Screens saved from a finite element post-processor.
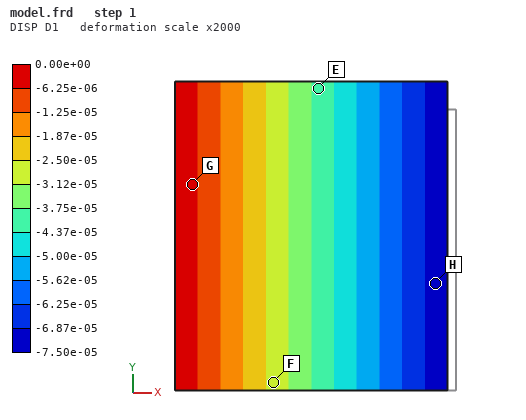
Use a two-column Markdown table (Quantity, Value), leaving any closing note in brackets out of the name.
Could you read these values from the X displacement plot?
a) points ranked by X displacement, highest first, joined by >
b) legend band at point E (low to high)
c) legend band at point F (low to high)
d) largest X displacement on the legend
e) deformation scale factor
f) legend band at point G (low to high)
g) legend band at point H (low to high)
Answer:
| Quantity | Value |
|---|---|
| points ranked by X displacement, highest first, joined by > | G > F > E > H |
| legend band at point E | -4.37e-05 to -3.75e-05 |
| legend band at point F | -3.12e-05 to -2.50e-05 |
| largest X displacement on the legend | 0.00e+00 |
| deformation scale factor | 2000 |
| legend band at point G | -6.25e-06 to 0.00e+00 |
| legend band at point H | -7.50e-05 to -6.87e-05 |
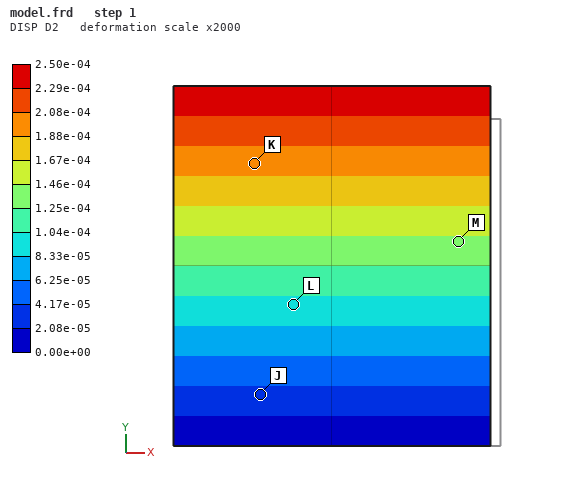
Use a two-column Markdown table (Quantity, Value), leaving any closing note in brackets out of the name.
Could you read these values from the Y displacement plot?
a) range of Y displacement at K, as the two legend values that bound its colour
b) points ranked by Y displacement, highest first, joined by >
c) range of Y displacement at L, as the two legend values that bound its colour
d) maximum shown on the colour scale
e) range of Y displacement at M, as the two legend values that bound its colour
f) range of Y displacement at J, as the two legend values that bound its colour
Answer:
| Quantity | Value |
|---|---|
| range of Y displacement at K, as the two legend values that bound its colour | 1.88e-04 to 2.08e-04 |
| points ranked by Y displacement, highest first, joined by > | K > M > L > J |
| range of Y displacement at L, as the two legend values that bound its colour | 8.33e-05 to 1.04e-04 |
| maximum shown on the colour scale | 2.50e-04 |
| range of Y displacement at M, as the two legend values that bound its colour | 1.25e-04 to 1.46e-04 |
| range of Y displacement at J, as the two legend values that bound its colour | 2.08e-05 to 4.17e-05 |
